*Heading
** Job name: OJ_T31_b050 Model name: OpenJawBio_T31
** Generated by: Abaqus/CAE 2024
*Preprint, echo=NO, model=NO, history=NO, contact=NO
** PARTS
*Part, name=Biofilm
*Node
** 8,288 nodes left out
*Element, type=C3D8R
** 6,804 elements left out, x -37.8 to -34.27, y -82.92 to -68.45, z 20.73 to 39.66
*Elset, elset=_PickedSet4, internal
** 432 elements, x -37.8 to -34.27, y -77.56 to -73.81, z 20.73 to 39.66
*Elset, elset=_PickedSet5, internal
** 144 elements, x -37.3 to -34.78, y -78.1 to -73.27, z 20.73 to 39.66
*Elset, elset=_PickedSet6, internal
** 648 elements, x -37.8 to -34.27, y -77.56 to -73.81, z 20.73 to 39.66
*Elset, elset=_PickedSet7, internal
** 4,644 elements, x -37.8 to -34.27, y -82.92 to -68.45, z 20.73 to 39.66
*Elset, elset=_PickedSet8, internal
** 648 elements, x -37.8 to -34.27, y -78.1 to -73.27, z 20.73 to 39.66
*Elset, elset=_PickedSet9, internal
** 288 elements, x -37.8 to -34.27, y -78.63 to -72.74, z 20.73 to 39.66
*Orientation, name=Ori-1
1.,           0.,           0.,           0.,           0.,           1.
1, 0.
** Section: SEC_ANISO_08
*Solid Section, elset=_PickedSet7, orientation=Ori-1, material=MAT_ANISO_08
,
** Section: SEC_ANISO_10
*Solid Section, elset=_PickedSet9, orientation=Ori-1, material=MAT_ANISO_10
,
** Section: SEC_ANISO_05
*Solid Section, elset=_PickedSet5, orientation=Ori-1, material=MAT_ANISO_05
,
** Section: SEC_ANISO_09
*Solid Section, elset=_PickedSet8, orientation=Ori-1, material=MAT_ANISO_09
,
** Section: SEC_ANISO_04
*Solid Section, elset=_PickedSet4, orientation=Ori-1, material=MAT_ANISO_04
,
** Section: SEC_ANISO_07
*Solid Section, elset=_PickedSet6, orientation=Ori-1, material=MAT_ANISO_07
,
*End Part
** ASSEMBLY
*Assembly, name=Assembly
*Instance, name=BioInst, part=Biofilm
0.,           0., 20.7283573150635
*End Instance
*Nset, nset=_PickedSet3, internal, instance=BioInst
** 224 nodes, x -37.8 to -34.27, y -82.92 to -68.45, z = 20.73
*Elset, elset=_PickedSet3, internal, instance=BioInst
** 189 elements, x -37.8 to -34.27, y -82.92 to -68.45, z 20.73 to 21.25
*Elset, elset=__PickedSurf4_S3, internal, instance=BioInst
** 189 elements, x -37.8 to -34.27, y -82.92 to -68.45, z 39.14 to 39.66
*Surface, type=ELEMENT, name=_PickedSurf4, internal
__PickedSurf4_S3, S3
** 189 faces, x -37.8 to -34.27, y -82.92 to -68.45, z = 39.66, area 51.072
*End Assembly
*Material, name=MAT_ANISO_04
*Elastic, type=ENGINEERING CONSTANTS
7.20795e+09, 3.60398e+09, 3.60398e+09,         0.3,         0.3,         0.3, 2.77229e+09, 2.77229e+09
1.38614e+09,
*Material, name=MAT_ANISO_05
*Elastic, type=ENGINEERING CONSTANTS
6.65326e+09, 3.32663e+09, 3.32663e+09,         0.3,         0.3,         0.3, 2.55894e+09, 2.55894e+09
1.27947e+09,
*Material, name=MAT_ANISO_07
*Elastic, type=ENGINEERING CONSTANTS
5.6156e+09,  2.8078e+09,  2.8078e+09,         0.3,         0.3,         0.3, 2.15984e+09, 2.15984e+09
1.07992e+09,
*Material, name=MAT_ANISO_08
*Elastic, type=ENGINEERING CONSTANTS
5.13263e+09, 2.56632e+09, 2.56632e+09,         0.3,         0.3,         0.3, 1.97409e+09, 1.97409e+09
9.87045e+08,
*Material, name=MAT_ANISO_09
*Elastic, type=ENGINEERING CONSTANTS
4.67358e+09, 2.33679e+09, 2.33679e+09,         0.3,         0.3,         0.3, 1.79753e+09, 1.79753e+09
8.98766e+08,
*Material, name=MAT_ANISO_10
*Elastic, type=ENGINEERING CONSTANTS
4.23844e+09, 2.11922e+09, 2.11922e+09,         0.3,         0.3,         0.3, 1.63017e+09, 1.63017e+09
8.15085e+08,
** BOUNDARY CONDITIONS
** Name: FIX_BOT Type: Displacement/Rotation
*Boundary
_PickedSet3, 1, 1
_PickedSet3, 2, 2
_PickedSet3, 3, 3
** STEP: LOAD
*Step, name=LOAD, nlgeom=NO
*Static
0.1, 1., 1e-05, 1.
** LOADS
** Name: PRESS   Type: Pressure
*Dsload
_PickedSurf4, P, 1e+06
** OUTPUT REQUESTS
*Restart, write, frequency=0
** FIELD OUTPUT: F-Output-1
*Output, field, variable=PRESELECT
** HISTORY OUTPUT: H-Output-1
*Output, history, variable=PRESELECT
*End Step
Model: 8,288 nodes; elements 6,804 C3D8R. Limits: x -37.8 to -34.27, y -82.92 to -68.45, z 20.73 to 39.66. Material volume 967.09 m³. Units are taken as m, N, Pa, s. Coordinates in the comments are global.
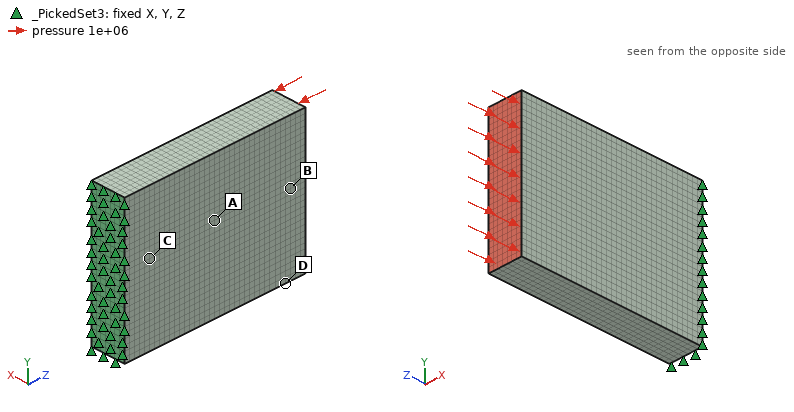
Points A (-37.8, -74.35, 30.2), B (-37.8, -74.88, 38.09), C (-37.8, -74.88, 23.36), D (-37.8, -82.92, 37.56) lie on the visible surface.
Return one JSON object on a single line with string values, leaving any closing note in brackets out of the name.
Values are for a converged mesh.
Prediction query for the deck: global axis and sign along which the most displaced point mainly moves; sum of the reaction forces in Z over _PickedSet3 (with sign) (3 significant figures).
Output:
{"global axis and sign along which the most displaced point mainly moves": "-Z", "sum of the reaction forces in Z over _PickedSet3 (with sign)": "5.11e+07 N"}
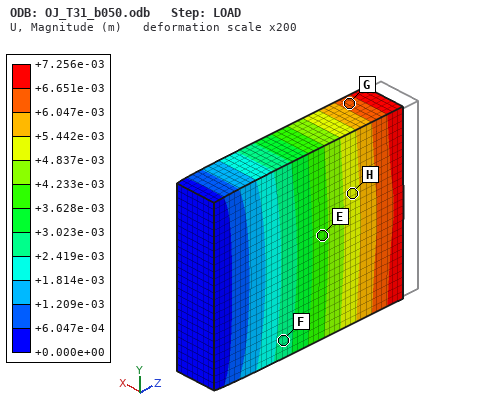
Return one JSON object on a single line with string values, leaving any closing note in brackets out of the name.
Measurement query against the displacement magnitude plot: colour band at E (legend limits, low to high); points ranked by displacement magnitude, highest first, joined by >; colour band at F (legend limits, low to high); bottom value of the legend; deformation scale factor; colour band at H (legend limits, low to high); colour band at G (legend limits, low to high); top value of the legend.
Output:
{"colour band at E": "+3.628e-03 to +4.233e-03 m", "points ranked by displacement magnitude, highest first, joined by >": "G > H > E > F", "colour band at F": "+2.419e-03 to +3.023e-03 m", "bottom value of the legend": "+0.000e+00 m", "deformation scale factor": "200", "colour band at H": "+4.837e-03 to +5.442e-03 m", "colour band at G": "+6.047e-03 to +6.651e-03 m", "top value of the legend": "+7.256e-03 m"}
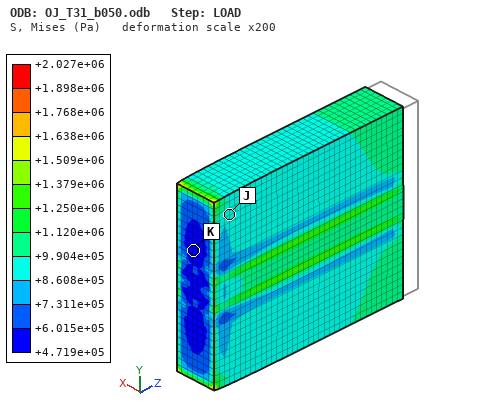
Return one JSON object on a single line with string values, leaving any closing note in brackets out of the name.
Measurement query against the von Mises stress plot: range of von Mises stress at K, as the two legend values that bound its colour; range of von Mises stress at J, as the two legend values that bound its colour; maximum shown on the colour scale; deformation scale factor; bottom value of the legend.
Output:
{"range of von Mises stress at K, as the two legend values that bound its colour": "+4.719e+05 to +6.015e+05 Pa", "range of von Mises stress at J, as the two legend values that bound its colour": "+8.608e+05 to +9.904e+05 Pa", "maximum shown on the colour scale": "+2.027e+06 Pa", "deformation scale factor": "200", "bottom value of the legend": "+4.719e+05 Pa"}
